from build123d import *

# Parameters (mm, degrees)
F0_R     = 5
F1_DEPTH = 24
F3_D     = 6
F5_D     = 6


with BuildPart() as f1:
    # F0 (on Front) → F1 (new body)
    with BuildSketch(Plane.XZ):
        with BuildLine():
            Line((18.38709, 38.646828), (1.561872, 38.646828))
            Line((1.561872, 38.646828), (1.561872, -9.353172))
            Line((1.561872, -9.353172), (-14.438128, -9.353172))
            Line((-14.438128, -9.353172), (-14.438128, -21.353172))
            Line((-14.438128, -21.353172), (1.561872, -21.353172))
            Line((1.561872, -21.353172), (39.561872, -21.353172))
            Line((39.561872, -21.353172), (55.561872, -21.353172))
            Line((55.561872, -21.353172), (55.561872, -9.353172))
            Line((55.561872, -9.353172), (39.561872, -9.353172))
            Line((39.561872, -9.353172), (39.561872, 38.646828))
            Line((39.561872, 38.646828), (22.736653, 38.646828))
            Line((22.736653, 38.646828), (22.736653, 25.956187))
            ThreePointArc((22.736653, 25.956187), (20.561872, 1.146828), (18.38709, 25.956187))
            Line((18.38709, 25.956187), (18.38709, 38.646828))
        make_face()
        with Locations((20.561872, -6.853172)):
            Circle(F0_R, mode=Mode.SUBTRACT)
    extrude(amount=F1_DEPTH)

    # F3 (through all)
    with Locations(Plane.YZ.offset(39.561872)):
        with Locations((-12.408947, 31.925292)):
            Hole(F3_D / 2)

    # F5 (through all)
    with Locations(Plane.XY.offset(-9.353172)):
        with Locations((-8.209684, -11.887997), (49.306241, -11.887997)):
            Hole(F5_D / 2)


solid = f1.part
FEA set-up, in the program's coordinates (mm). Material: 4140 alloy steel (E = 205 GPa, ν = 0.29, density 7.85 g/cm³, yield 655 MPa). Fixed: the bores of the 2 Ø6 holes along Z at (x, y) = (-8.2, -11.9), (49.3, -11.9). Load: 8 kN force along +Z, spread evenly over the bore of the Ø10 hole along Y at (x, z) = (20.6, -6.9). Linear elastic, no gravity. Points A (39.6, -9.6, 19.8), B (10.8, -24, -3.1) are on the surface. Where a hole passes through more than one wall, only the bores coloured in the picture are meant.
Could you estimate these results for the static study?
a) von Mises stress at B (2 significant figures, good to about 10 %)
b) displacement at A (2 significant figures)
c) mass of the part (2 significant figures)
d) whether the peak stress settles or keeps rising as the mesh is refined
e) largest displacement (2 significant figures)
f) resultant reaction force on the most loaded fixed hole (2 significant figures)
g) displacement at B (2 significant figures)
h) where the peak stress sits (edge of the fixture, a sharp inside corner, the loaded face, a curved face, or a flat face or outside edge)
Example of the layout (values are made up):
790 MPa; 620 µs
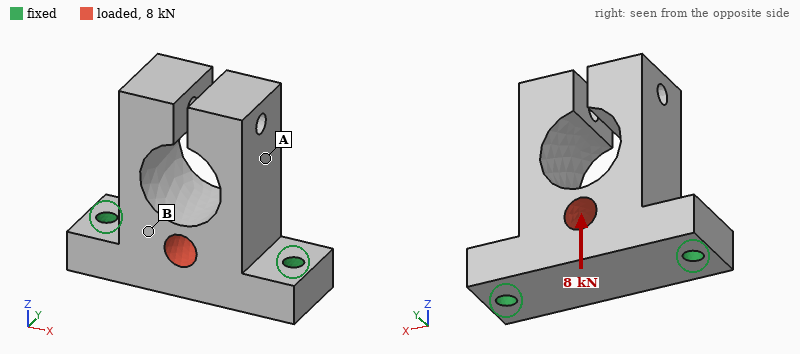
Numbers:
26 MPa; 6.7 µm; 370 g; keeps rising; 11 µm; 4.3 kN; 6.6 µm; edge of the fixture
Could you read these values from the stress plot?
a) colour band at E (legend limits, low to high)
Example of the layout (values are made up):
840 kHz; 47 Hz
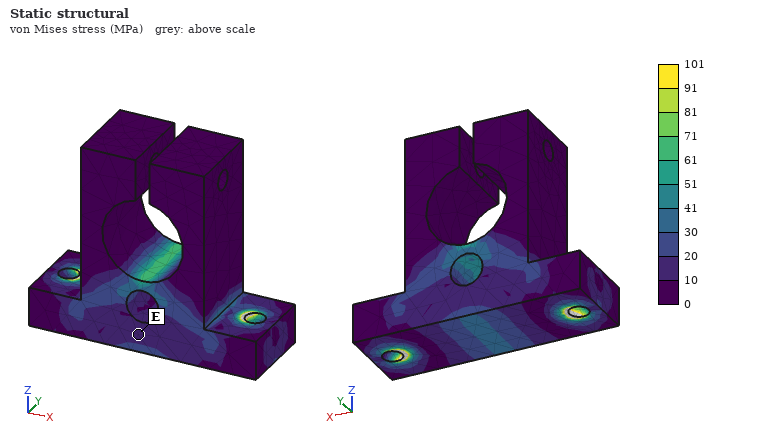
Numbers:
10 to 20 MPa
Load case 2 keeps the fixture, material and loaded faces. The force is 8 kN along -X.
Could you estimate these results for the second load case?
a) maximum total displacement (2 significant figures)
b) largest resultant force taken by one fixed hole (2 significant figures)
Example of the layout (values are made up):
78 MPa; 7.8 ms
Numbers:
7.2 µm; 4.2 kN
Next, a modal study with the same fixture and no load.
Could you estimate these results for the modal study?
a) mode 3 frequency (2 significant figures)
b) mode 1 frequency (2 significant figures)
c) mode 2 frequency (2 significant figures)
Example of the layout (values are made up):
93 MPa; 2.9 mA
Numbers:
2900 Hz; 2800 Hz; 2900 Hz
